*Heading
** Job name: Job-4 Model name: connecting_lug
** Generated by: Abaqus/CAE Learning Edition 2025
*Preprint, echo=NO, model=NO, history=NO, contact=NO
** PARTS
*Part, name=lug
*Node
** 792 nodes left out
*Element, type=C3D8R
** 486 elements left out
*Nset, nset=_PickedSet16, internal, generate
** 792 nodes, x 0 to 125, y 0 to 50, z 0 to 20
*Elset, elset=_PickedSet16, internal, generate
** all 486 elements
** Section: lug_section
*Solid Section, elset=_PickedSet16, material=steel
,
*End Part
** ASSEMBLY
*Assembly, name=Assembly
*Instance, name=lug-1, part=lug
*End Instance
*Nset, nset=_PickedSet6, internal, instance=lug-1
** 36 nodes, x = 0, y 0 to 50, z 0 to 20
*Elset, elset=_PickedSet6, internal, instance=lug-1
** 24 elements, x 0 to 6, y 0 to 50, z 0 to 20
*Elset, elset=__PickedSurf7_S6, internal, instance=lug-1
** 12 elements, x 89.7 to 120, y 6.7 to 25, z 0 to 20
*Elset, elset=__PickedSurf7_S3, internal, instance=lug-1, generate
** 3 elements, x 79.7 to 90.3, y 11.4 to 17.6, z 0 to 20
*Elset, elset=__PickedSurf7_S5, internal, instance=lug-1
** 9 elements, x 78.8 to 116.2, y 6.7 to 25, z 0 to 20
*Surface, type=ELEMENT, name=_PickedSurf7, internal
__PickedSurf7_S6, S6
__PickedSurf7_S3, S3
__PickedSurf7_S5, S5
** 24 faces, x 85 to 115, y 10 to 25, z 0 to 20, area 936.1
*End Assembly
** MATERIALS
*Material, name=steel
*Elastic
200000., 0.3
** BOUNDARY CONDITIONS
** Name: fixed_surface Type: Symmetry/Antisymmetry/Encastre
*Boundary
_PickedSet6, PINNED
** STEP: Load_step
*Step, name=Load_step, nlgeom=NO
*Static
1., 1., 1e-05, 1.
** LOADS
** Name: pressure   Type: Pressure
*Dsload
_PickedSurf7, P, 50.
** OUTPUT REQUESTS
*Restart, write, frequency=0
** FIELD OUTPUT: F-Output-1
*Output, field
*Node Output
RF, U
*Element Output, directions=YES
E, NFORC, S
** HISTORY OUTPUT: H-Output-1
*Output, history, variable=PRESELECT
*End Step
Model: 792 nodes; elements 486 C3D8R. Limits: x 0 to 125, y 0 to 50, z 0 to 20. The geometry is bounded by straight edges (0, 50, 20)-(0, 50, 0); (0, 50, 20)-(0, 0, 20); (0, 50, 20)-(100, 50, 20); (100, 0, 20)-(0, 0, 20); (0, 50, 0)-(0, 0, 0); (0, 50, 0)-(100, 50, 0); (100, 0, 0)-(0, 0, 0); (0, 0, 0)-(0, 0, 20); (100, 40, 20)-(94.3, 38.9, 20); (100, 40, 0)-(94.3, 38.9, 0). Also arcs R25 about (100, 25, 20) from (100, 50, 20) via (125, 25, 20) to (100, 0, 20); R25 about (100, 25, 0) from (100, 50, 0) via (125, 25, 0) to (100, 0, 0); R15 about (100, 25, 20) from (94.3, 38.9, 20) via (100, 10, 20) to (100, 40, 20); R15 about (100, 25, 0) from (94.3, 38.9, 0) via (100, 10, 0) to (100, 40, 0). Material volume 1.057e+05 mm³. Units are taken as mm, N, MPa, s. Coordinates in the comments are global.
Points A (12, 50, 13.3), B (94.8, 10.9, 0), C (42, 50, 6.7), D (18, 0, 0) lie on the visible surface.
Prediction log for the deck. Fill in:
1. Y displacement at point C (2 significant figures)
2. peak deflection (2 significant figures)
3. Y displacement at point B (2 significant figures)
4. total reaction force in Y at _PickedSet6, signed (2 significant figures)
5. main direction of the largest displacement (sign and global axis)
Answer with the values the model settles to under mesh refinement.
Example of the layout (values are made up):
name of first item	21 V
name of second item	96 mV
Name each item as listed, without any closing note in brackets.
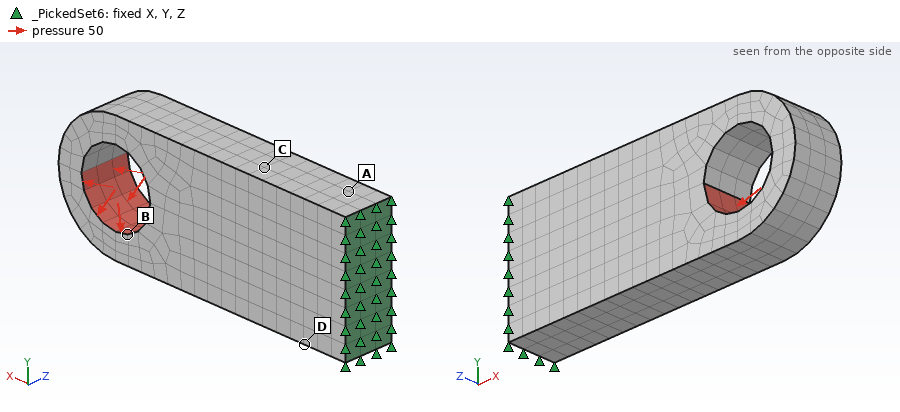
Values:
Y displacement at point C	-0.074 mm
peak deflection	0.42 mm
Y displacement at point B	-0.28 mm
total reaction force in Y at _PickedSet6, signed	30000 N
main direction of the largest displacement	-Y
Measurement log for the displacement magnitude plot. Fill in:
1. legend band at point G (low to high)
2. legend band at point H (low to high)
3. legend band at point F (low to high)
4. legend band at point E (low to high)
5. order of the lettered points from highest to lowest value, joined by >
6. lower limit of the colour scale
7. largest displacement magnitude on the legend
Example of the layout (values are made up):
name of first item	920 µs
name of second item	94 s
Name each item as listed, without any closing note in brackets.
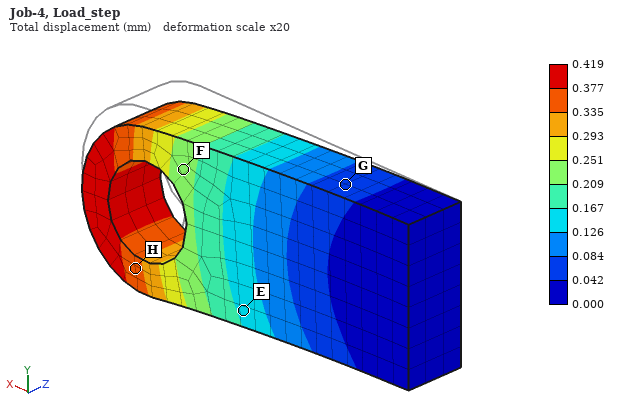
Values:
legend band at point G	0.042 to 0.084 mm
legend band at point H	0.335 to 0.377 mm
legend band at point F	0.209 to 0.251 mm
legend band at point E	0.126 to 0.167 mm
order of the lettered points from highest to lowest value, joined by >	H > F > E > G
lower limit of the colour scale	0.000 mm
largest displacement magnitude on the legend	0.419 mm
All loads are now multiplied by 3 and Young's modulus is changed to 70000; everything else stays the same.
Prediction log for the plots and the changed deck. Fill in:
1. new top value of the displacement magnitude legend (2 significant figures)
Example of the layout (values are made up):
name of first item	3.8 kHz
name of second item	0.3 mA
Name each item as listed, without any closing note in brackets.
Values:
new top value of the displacement magnitude legend	3.6 mm
